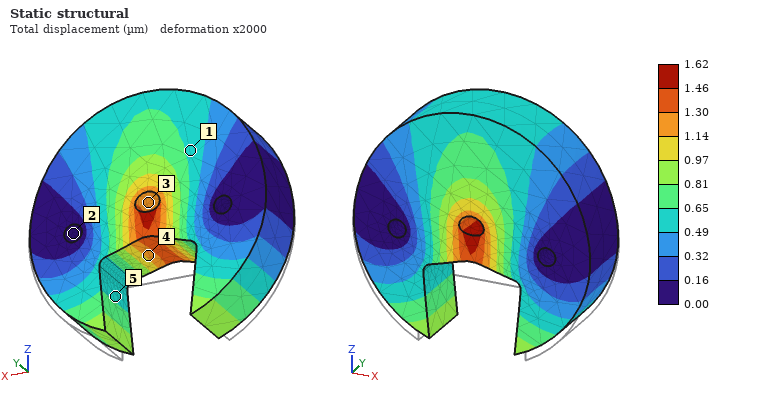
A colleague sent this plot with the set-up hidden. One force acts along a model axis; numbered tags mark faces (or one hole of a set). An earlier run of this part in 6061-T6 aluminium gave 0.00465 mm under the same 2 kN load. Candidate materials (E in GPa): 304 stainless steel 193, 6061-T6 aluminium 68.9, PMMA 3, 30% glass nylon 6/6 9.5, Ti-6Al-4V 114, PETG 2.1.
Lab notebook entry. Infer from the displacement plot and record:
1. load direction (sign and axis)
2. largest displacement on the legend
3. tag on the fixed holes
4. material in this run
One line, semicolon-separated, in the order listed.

+Z; 1.62 µm; 2; 304 stainless steel
